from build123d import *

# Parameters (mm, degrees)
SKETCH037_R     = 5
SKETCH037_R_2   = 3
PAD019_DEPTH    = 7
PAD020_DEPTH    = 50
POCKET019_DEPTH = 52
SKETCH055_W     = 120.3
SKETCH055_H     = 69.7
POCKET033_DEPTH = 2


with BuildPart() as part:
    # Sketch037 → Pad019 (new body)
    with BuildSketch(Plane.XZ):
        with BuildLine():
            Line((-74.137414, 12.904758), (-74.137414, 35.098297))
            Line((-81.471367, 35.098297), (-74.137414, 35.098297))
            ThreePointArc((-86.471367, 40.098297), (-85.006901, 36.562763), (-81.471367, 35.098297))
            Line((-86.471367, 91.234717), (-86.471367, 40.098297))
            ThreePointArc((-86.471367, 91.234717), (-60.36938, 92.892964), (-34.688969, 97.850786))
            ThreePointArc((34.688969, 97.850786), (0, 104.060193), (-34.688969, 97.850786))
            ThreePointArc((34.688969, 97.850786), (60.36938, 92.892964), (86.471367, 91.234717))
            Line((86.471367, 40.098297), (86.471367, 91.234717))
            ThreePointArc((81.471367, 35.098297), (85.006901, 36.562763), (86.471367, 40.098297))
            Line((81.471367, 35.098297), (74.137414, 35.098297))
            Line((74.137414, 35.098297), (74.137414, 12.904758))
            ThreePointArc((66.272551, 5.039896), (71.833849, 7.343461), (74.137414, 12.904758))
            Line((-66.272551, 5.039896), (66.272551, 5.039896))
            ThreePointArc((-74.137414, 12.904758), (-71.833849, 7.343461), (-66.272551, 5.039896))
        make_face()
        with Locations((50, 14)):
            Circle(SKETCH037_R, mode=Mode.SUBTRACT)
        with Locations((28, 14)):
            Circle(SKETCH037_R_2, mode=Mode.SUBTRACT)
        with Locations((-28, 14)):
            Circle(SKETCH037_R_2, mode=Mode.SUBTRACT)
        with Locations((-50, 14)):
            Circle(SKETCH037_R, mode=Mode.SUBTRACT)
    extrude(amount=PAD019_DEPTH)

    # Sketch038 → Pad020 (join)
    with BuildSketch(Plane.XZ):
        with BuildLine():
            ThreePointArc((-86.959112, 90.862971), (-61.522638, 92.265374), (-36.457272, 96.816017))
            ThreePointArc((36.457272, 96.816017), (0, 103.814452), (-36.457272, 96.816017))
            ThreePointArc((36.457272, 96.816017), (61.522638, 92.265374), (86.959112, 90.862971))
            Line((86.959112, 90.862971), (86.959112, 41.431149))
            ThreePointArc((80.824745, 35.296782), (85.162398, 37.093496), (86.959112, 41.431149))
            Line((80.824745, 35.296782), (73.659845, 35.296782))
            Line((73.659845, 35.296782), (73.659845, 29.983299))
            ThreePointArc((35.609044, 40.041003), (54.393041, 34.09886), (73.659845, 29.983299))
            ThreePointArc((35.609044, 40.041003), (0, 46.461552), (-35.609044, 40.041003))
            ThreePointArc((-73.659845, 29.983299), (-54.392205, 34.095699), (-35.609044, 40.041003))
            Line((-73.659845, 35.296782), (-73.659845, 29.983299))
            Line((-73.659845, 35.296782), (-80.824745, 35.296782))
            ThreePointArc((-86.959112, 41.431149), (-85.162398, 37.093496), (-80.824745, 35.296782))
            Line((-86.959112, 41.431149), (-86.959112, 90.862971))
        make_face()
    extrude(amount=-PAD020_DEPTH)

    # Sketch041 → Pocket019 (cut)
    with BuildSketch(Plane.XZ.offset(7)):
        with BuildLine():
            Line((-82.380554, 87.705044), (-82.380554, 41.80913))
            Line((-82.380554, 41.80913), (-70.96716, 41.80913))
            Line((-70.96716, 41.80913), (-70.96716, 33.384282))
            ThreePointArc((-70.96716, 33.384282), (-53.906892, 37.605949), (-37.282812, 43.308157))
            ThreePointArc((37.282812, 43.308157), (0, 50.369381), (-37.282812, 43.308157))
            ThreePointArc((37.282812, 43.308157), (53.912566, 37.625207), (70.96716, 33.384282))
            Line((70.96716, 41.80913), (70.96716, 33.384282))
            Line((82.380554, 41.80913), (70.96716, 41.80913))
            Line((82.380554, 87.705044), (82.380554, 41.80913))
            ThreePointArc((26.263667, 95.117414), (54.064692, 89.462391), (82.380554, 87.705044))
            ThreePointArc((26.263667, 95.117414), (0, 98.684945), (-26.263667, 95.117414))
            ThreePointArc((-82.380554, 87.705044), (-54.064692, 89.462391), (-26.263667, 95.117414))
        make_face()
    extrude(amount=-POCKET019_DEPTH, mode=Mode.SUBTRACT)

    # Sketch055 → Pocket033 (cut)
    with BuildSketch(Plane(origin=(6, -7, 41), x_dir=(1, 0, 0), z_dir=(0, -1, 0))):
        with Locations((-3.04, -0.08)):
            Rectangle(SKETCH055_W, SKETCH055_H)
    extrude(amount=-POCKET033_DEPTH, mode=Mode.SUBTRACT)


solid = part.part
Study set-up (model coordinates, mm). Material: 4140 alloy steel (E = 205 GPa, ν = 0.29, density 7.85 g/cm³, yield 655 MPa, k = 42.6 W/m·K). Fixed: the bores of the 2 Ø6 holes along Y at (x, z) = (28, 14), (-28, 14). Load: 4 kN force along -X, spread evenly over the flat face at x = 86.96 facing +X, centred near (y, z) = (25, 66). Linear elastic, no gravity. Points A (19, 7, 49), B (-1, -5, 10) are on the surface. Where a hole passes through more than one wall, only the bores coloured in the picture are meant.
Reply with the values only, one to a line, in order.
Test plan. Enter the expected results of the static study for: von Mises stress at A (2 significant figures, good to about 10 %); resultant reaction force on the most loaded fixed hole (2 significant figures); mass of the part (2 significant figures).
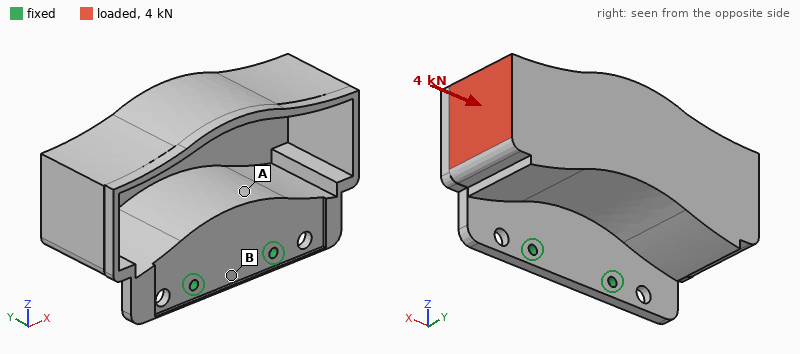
41 MPa
4.3 kN
1.4 kg
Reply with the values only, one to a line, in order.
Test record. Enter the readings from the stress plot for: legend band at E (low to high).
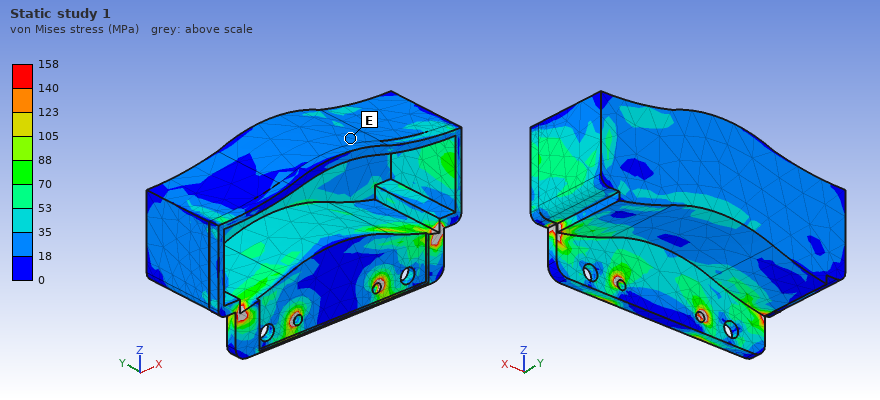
18 to 35 MPa
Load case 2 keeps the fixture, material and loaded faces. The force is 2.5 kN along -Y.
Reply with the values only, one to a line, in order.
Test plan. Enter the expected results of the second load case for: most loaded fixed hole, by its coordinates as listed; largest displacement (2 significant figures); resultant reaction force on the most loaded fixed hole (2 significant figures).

(28, 14)
2.0 mm
4.4 kN
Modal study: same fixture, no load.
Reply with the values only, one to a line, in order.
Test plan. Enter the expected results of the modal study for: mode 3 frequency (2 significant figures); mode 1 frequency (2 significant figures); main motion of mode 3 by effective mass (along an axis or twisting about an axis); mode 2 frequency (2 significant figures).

630 Hz
220 Hz
along X
370 Hz
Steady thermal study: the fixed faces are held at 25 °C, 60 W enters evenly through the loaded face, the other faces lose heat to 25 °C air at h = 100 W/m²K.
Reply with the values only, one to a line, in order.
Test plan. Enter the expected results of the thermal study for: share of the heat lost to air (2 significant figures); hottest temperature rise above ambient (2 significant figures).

98 %
62 K
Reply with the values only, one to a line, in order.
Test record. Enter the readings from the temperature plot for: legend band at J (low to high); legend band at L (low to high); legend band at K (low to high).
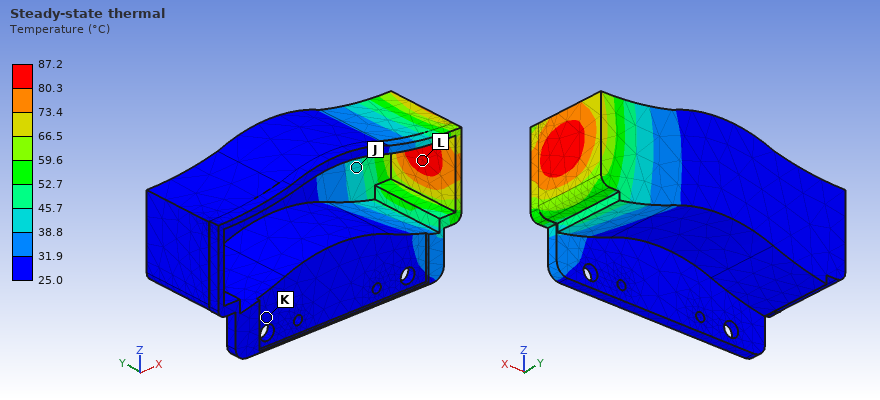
38.8 to 45.7 °C
80.3 to 87.2 °C
25.0 to 31.9 °C
